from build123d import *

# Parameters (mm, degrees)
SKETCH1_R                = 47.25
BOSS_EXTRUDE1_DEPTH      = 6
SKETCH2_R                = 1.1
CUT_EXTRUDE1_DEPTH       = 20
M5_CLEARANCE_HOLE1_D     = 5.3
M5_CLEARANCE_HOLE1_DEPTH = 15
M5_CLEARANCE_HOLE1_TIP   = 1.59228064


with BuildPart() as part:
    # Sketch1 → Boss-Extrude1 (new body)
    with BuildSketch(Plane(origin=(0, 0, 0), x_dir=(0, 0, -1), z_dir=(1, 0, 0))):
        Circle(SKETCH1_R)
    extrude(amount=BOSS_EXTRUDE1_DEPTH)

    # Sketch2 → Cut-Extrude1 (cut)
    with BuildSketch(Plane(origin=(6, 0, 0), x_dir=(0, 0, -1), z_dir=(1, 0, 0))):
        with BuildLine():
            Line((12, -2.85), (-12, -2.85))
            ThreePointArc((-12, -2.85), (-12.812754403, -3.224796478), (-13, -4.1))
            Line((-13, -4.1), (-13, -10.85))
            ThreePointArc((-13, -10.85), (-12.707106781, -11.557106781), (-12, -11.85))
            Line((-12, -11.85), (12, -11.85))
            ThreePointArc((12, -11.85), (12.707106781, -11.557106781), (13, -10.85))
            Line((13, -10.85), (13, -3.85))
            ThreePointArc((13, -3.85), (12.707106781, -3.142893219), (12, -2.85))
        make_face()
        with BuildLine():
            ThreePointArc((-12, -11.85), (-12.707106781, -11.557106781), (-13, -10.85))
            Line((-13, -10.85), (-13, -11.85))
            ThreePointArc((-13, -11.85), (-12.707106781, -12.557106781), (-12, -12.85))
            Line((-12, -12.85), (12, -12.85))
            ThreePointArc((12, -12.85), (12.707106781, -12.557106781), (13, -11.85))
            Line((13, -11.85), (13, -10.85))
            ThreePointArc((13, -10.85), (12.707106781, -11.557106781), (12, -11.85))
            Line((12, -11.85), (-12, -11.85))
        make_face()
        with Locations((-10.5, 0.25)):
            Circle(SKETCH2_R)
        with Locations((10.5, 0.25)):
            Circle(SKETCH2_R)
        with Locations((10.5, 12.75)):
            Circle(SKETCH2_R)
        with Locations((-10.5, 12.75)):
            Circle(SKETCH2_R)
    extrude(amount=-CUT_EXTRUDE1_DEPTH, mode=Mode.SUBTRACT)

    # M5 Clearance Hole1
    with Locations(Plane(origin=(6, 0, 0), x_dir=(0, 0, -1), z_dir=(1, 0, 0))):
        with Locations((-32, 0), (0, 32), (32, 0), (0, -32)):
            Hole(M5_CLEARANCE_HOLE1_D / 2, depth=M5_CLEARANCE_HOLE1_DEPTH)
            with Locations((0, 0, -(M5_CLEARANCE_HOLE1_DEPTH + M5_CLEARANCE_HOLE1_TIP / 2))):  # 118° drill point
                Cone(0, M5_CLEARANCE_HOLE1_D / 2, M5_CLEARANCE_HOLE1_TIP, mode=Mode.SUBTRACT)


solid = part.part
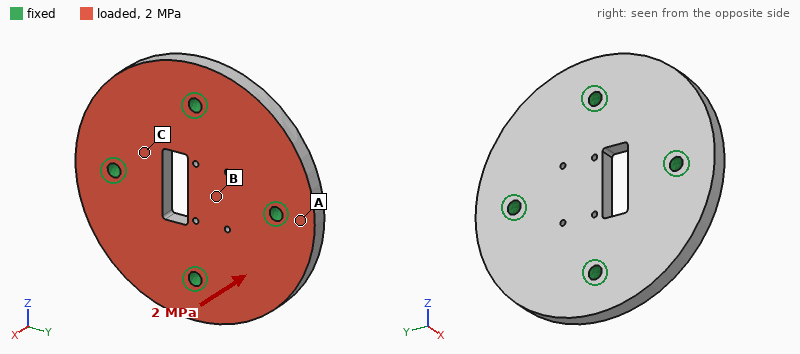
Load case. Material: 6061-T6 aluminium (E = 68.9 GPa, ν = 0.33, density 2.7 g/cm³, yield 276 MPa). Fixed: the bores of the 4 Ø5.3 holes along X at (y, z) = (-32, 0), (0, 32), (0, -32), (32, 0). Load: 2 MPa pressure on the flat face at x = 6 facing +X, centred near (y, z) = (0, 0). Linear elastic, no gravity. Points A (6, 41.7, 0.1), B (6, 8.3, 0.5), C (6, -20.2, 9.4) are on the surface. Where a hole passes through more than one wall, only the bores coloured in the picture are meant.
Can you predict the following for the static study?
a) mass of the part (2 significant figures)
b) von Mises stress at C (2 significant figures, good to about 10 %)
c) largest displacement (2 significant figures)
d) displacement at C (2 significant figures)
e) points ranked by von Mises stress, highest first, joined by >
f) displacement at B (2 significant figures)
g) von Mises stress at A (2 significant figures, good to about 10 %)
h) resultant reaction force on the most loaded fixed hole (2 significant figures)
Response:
110 g
28 MPa
73 µm
18 µm
A > C > B
27 µm
53 MPa
3.4 kN
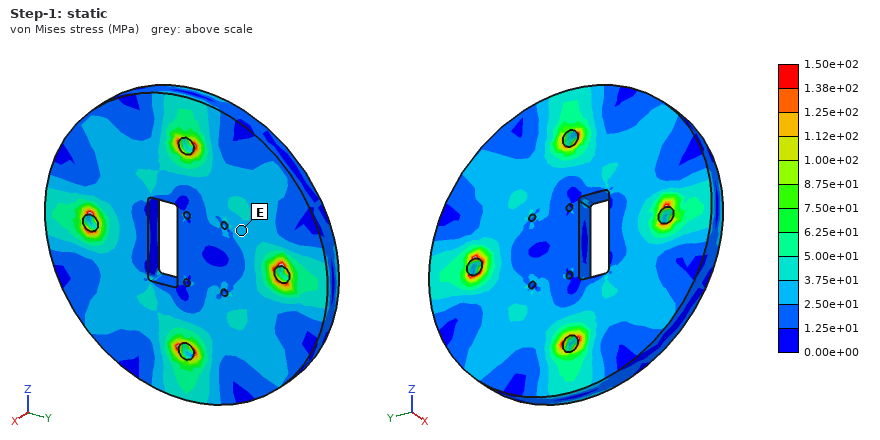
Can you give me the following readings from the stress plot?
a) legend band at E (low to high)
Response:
2.50e+01 to 3.75e+01 MPa
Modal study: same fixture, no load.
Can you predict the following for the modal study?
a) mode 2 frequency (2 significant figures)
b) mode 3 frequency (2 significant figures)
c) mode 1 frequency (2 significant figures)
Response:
7800 Hz
7800 Hz
7100 Hz
